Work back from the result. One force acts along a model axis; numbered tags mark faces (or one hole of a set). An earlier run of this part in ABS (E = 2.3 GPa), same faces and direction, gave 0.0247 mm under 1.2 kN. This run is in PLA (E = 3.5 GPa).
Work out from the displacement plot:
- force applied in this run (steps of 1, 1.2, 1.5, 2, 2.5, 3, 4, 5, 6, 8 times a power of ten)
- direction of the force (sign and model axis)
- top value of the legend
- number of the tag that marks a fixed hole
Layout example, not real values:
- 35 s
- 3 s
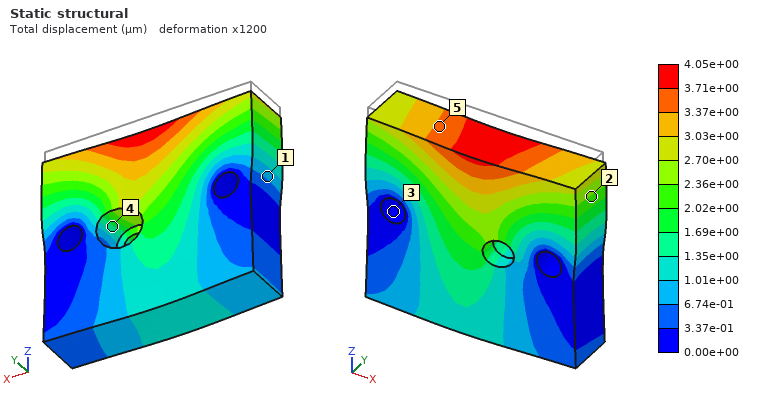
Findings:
- 300 N
- -Z
- 4.05e+00 µm
- 3
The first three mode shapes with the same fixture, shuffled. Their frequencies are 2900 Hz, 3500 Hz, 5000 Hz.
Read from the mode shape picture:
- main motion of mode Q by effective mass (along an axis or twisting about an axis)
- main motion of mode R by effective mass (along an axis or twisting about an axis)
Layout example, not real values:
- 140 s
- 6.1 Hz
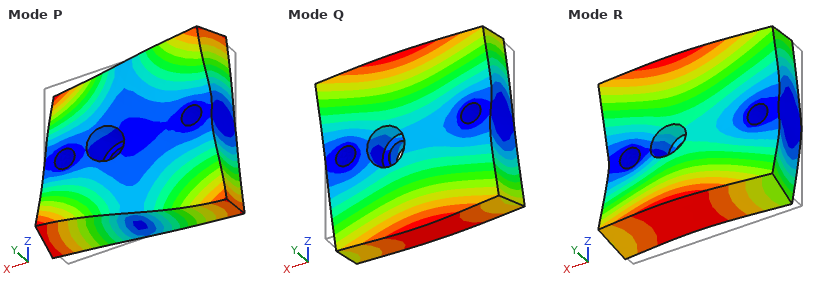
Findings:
- twisting about X
- along Y
